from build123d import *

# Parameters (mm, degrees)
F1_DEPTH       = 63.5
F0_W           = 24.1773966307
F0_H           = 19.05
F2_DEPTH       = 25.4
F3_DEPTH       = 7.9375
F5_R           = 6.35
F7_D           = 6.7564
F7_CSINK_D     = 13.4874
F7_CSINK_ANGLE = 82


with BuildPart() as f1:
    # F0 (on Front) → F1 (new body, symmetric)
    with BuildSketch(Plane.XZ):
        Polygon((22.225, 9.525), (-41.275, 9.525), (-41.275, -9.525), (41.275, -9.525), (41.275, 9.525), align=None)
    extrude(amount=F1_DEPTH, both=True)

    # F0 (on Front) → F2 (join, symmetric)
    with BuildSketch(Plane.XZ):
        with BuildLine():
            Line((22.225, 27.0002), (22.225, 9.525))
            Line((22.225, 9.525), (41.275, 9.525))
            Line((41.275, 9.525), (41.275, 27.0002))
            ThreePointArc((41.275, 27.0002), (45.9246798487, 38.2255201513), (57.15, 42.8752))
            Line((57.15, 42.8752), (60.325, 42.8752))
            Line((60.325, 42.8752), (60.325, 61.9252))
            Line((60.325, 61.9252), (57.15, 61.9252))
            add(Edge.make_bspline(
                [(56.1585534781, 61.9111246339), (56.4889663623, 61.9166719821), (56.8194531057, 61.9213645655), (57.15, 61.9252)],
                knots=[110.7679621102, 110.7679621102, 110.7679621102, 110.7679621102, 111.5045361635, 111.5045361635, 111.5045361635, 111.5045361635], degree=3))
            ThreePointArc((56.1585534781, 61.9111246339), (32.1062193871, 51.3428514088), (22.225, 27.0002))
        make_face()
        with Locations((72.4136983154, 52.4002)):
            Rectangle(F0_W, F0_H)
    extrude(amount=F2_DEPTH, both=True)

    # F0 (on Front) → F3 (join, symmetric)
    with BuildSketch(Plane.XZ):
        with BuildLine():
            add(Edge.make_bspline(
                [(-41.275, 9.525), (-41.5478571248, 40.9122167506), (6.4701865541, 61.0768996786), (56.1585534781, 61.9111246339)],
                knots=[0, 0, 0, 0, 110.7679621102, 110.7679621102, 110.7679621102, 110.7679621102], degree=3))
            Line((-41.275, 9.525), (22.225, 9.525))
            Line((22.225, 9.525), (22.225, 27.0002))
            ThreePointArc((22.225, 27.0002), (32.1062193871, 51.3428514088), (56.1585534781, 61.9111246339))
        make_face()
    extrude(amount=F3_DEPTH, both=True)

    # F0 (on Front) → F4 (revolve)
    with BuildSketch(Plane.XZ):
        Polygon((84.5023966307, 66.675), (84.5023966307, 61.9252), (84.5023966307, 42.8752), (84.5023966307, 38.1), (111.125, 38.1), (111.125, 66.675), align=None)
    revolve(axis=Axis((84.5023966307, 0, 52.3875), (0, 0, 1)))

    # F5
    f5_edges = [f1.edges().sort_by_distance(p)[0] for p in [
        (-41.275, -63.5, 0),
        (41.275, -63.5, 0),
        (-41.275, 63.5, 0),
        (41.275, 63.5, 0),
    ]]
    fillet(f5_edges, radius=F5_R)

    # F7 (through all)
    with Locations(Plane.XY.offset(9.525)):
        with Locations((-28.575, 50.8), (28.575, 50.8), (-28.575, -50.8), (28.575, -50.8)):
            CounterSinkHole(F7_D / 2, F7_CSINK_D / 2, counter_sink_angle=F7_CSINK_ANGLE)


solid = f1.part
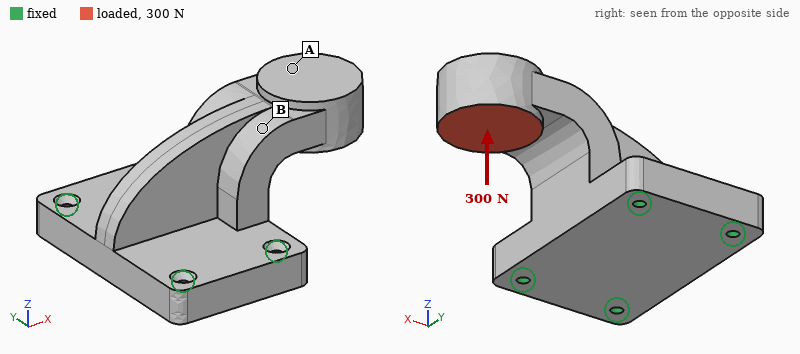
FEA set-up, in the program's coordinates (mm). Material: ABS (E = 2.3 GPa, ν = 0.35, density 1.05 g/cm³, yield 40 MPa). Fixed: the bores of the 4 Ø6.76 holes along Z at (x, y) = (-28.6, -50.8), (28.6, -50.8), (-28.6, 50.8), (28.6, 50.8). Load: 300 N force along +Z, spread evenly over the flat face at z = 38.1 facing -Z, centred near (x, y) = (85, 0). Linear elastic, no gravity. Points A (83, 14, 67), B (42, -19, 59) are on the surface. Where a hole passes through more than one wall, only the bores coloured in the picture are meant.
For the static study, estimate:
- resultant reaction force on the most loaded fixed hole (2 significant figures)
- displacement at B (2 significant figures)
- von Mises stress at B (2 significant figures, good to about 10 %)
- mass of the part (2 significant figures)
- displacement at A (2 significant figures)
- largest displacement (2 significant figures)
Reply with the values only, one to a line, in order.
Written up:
300 N
0.18 mm
2.1 MPa
380 g
0.45 mm
0.65 mm
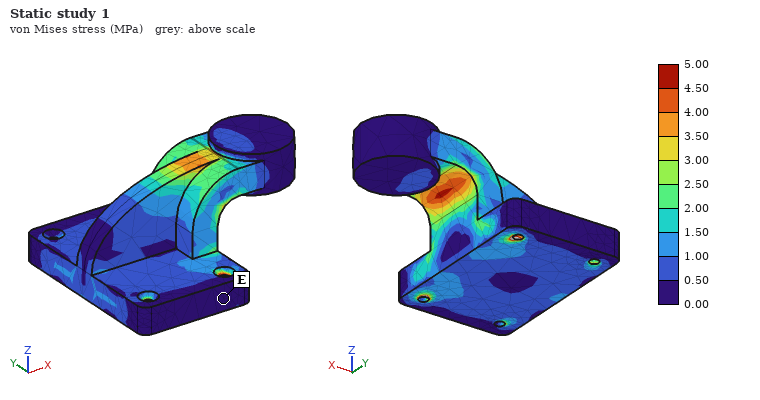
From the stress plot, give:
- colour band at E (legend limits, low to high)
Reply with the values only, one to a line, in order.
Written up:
0.00 to 0.50 MPa
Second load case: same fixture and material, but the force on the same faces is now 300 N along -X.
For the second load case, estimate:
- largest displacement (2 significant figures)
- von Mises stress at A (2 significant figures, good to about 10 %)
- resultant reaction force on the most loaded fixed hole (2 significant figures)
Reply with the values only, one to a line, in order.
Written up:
81 µm
0.24 MPa
140 N
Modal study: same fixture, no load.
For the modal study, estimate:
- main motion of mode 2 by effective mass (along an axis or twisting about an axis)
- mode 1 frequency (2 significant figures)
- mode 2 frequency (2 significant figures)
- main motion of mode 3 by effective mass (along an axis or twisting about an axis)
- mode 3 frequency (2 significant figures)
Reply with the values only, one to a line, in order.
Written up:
along Y
460 Hz
530 Hz
along X
1100 Hz
